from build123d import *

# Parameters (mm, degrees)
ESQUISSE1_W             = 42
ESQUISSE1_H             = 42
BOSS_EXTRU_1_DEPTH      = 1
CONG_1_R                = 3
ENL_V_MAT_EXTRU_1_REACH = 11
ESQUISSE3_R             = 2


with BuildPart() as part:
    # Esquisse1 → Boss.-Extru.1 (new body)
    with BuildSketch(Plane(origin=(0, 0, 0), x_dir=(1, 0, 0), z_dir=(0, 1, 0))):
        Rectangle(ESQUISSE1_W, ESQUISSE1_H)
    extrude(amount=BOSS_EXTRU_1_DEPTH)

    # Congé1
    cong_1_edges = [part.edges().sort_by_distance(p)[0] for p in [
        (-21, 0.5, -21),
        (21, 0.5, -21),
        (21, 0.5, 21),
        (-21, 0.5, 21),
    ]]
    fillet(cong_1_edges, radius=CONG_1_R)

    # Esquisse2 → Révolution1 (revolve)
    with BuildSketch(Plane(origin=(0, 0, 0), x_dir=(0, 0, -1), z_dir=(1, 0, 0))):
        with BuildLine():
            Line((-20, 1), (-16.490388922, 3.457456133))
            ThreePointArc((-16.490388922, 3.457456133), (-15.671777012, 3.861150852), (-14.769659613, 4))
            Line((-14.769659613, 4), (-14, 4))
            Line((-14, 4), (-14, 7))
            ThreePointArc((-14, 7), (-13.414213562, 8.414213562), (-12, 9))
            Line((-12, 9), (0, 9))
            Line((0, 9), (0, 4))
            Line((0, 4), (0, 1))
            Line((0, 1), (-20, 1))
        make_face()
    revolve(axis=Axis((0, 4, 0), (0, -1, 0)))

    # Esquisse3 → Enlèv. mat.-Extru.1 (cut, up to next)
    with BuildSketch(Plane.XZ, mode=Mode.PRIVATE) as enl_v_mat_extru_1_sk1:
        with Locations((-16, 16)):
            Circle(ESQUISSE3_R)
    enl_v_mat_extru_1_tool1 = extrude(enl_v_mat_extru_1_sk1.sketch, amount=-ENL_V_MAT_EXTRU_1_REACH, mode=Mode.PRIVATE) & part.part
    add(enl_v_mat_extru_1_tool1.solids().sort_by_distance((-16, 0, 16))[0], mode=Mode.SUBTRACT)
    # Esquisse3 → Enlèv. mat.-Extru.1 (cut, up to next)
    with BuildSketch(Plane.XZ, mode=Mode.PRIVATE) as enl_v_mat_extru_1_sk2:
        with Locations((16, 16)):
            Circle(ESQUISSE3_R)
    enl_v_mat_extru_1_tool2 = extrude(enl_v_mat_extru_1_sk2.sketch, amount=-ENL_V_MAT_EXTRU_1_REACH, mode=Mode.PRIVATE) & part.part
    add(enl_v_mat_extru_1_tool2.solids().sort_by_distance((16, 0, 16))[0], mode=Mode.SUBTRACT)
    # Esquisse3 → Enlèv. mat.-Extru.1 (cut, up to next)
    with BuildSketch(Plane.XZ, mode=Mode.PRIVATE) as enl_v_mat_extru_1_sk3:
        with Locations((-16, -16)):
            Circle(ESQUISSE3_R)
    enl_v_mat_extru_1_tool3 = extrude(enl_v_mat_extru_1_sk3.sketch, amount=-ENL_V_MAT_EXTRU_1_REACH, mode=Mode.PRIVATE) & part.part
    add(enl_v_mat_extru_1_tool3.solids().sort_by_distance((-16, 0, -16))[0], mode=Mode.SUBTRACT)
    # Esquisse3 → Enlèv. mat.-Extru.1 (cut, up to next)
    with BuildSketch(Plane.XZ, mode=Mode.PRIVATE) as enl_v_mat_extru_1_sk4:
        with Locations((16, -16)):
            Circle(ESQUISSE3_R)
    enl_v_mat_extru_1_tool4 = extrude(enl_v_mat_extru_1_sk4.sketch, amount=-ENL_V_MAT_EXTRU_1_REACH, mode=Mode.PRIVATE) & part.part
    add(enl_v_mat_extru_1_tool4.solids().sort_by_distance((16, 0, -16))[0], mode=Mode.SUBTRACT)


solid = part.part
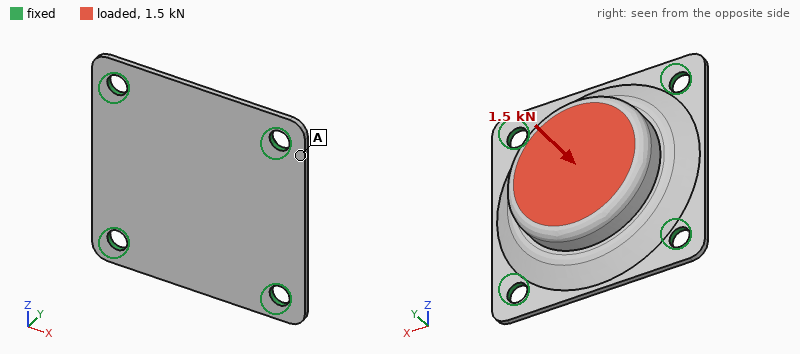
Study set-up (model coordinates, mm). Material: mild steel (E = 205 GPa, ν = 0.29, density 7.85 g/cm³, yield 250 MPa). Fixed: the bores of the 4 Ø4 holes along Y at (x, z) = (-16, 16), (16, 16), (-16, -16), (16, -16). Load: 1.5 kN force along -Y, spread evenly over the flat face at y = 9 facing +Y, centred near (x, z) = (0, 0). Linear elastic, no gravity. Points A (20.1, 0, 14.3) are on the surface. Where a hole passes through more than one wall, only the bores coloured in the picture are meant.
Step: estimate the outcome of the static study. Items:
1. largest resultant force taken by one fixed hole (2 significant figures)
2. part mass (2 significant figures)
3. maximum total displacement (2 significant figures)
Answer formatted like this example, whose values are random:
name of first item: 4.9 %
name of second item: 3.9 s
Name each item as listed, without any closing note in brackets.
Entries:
largest resultant force taken by one fixed hole: 660 N
part mass: 61 g
maximum total displacement: 9.2 µm
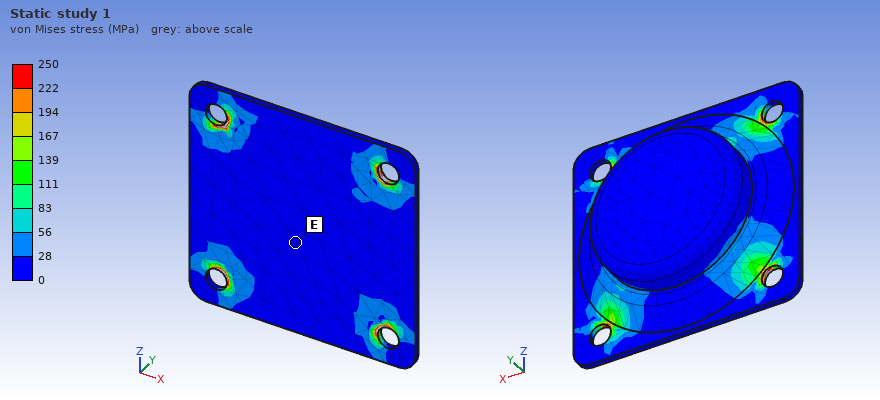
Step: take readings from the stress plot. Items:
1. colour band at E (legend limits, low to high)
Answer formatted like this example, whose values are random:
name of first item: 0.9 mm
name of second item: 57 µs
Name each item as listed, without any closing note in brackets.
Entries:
colour band at E: 0 to 28 MPa
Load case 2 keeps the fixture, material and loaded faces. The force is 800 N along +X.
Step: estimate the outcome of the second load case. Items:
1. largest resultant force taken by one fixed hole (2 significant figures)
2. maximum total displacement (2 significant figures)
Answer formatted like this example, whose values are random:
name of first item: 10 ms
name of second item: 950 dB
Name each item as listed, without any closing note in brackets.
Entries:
largest resultant force taken by one fixed hole: 270 N
maximum total displacement: 3.5 µm
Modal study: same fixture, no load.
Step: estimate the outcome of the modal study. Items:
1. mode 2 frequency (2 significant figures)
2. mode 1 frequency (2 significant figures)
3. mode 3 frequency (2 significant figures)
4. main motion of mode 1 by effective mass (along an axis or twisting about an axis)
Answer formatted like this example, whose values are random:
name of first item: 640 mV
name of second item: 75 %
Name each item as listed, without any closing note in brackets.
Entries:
mode 2 frequency: 13 kHz
mode 1 frequency: 8900 Hz
mode 3 frequency: 13 kHz
main motion of mode 1 by effective mass: along Y
